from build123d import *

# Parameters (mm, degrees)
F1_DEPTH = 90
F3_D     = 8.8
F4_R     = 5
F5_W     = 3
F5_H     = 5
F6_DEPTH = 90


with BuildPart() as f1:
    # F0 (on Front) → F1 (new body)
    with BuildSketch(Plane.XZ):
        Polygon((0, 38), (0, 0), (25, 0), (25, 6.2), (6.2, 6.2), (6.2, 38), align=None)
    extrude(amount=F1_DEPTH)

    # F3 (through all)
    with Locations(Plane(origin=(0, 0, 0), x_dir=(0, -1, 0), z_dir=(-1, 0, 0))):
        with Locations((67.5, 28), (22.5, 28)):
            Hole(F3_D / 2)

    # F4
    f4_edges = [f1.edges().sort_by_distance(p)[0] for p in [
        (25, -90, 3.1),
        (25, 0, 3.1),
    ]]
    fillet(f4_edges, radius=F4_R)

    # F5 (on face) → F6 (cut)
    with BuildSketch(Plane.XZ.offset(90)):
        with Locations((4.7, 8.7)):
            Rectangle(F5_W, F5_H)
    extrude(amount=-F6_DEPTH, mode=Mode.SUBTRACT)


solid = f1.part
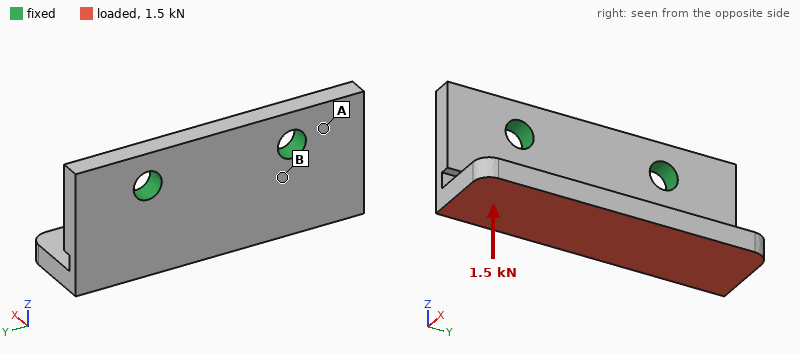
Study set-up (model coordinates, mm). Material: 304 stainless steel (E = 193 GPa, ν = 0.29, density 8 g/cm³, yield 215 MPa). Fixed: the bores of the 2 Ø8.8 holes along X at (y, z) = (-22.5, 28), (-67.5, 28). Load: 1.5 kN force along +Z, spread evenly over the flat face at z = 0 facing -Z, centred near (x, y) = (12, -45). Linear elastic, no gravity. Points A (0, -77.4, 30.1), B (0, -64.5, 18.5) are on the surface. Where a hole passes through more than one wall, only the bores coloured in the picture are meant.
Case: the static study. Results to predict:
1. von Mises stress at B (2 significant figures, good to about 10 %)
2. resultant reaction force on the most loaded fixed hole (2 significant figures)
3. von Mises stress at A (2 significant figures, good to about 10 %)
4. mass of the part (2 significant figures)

23 MPa
750 N
8.0 MPa
240 g
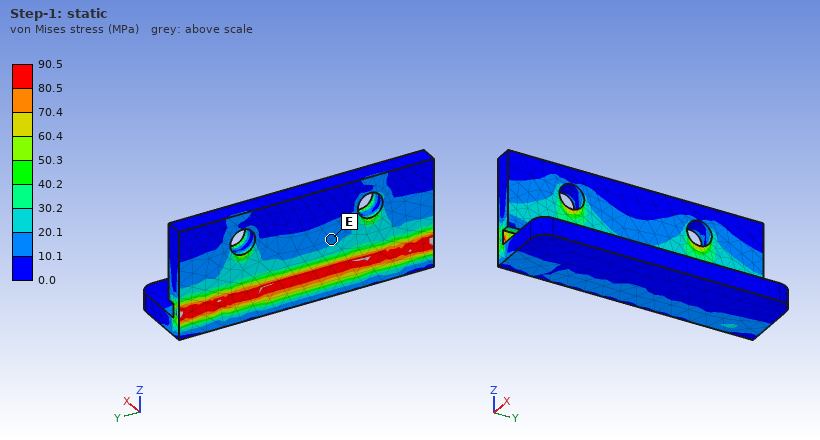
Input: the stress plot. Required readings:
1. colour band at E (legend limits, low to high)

10.1 to 20.1 MPa
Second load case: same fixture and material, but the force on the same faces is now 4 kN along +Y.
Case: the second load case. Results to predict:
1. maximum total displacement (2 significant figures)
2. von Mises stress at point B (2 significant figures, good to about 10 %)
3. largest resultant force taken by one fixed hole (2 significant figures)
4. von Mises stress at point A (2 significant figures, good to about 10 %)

34 µm
35 MPa
2.9 kN
38 MPa
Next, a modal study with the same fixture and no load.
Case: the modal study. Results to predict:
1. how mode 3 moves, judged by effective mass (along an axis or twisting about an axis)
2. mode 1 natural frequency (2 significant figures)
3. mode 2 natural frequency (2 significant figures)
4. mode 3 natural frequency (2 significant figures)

along X
2200 Hz
3600 Hz
5600 Hz
